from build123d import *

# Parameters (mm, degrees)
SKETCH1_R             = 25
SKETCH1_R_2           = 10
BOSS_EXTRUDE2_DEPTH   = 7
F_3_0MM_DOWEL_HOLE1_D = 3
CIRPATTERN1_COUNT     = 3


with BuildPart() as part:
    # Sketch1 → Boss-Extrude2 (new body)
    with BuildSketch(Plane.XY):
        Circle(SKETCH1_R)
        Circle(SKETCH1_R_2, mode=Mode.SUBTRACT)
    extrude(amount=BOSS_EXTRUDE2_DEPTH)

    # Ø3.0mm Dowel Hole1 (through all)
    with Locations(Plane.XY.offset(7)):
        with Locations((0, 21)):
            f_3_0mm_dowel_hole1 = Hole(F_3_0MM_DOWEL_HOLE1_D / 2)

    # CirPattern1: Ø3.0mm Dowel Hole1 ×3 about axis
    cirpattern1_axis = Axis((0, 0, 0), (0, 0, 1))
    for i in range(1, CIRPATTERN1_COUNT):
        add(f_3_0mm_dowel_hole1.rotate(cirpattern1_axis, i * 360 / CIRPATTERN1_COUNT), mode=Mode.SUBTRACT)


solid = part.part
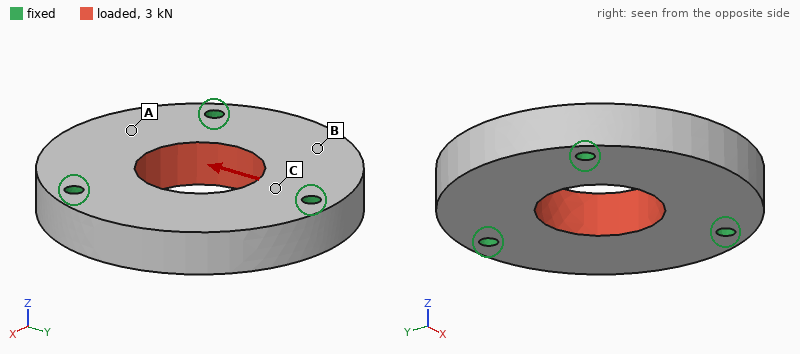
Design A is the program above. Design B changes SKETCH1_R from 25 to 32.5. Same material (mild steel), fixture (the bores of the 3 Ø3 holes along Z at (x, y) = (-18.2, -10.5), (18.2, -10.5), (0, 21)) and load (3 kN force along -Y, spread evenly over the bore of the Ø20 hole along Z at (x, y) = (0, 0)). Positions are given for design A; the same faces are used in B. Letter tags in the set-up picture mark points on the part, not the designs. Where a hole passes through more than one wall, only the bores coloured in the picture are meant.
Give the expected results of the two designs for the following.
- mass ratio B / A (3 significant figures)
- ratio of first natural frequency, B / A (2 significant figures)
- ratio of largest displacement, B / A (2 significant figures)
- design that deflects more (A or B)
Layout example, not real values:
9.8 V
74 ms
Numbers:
1.83
0.62
0.72
A
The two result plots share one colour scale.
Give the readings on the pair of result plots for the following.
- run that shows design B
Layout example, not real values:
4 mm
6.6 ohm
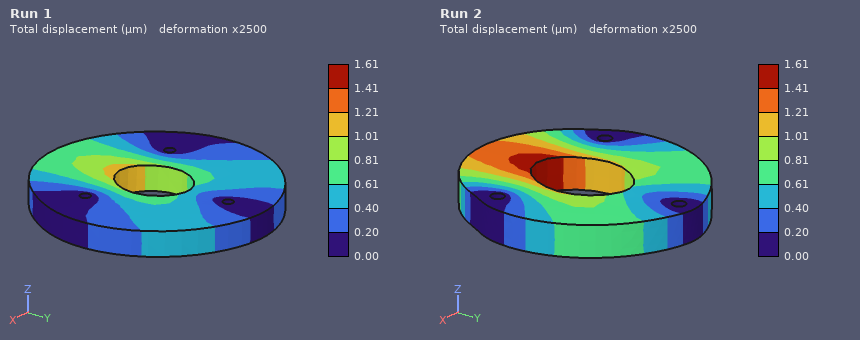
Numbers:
Run 1
